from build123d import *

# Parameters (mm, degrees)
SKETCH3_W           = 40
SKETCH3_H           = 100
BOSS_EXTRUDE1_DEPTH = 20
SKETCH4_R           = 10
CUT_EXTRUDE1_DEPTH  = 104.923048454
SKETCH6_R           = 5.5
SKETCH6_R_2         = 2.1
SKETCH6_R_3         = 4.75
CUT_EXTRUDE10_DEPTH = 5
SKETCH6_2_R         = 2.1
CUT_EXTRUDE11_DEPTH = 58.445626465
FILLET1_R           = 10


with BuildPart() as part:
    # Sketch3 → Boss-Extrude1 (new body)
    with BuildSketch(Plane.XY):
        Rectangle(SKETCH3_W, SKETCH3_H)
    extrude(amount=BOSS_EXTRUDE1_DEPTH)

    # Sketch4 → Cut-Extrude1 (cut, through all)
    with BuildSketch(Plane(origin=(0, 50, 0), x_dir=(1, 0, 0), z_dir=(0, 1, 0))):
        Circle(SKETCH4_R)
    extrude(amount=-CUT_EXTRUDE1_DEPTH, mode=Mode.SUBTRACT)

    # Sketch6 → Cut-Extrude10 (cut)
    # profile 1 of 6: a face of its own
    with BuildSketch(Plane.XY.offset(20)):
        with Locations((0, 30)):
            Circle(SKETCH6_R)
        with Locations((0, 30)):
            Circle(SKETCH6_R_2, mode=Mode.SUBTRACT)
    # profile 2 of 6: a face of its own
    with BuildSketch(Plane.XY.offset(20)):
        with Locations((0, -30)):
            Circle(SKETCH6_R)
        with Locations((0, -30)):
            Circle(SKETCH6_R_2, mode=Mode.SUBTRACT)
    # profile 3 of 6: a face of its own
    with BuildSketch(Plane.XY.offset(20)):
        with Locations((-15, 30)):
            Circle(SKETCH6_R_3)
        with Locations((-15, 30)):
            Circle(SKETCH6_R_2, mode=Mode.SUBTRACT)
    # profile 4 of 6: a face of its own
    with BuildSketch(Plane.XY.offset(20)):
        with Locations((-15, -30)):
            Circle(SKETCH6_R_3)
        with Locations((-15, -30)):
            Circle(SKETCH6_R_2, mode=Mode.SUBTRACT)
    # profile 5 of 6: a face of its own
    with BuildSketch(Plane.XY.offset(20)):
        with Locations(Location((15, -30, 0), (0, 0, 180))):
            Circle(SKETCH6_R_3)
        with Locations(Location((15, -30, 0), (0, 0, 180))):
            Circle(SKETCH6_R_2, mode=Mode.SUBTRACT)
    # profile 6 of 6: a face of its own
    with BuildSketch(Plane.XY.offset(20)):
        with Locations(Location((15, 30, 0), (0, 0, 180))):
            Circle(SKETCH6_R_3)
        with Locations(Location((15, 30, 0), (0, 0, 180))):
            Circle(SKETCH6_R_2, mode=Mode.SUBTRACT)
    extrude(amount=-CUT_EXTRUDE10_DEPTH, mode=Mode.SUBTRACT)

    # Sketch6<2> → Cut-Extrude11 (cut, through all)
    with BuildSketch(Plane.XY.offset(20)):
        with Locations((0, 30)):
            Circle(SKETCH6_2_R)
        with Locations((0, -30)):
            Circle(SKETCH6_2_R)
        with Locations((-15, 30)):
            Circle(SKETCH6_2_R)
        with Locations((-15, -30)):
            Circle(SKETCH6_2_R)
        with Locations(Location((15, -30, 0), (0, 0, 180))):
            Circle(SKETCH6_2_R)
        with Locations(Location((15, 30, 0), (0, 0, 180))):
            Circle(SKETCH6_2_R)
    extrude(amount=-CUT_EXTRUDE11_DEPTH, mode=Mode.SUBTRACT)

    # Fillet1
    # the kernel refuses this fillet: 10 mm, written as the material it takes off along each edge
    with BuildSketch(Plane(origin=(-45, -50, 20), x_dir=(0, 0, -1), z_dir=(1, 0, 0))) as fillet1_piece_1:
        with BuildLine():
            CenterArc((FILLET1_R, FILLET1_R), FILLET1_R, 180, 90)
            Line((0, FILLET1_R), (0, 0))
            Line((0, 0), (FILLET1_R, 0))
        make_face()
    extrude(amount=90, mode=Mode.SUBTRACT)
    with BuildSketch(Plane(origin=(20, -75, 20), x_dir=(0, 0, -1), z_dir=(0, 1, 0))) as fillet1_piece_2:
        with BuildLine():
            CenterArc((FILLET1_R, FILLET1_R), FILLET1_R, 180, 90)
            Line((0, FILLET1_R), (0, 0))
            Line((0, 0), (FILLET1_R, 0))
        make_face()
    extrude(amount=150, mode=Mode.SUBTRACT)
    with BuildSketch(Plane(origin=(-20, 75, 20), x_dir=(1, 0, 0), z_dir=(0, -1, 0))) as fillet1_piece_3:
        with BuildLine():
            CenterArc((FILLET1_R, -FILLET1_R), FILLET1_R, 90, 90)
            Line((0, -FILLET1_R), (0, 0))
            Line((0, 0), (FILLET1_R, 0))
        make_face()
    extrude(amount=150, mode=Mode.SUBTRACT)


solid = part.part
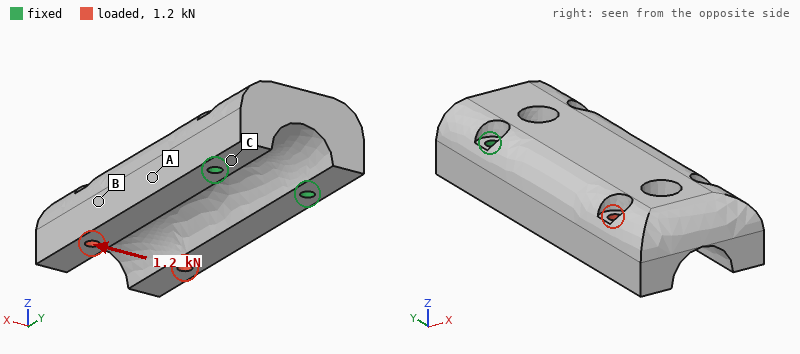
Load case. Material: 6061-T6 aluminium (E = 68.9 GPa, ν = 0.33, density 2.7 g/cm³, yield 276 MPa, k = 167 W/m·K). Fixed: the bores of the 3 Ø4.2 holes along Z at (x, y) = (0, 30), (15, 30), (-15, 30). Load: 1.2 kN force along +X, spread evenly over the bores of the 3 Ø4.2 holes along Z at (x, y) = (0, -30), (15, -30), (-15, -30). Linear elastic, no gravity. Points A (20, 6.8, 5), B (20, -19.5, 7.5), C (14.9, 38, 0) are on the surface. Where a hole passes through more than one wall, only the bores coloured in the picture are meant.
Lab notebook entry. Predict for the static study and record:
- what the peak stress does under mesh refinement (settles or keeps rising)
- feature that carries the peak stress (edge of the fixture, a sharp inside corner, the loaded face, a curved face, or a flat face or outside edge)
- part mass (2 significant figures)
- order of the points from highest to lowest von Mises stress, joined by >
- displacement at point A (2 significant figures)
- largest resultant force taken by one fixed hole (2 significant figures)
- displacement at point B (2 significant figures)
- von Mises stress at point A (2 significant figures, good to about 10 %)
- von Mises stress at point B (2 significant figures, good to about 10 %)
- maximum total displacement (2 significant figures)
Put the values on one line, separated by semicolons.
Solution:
keeps rising; edge of the fixture; 150 g; A > B > C; 11 µm; 2.3 kN; 28 µm; 12 MPa; 6.3 MPa; 49 µm
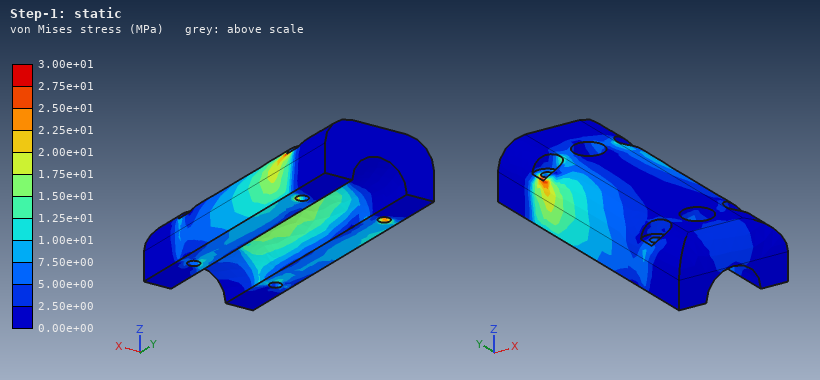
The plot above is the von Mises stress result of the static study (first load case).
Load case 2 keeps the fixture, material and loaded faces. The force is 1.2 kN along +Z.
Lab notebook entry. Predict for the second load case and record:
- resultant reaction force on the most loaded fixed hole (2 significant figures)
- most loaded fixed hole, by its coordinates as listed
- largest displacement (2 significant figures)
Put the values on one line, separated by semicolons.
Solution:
2.0 kN; (0, 30); 0.15 mm
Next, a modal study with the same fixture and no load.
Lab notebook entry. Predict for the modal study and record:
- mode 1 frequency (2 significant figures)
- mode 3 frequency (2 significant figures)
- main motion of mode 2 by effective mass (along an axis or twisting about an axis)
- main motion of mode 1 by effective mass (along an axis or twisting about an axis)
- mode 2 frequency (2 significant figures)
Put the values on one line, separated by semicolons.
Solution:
2100 Hz; 6100 Hz; along X; along Z; 3900 Hz
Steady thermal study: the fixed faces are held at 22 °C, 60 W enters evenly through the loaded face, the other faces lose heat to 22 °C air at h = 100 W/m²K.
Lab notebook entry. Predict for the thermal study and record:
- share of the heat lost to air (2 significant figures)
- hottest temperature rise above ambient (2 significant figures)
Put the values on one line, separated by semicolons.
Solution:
31 %; 30 K
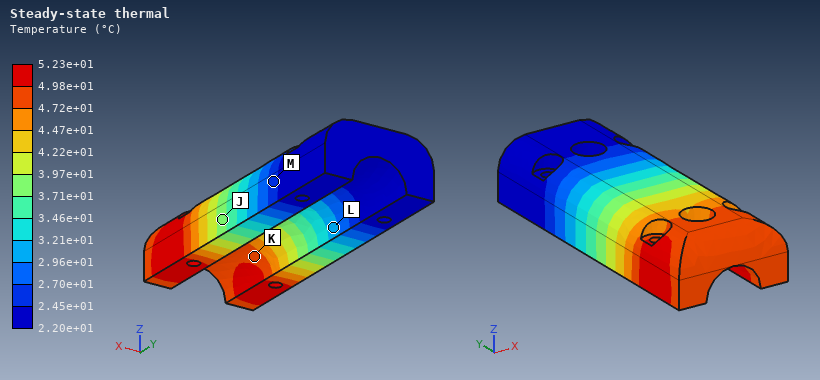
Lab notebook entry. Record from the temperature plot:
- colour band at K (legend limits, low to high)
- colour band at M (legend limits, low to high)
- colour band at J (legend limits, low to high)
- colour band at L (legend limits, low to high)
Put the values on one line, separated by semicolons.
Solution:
4.72e+01 to 4.98e+01 °C; 2.45e+01 to 2.70e+01 °C; 3.71e+01 to 3.97e+01 °C; 2.96e+01 to 3.21e+01 °C
